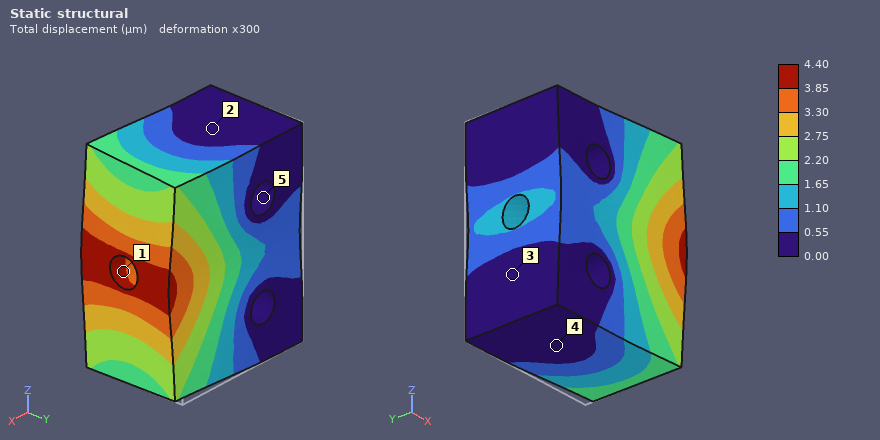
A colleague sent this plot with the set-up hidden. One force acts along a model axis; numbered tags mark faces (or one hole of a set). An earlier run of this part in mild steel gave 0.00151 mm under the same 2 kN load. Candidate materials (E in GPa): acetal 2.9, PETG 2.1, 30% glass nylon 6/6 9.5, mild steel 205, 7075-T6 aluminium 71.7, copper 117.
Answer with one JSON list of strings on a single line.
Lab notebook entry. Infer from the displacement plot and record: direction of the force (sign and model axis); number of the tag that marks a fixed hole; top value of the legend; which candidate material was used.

["-Y", "5", "4.40 µm", "7075-T6 aluminium"]
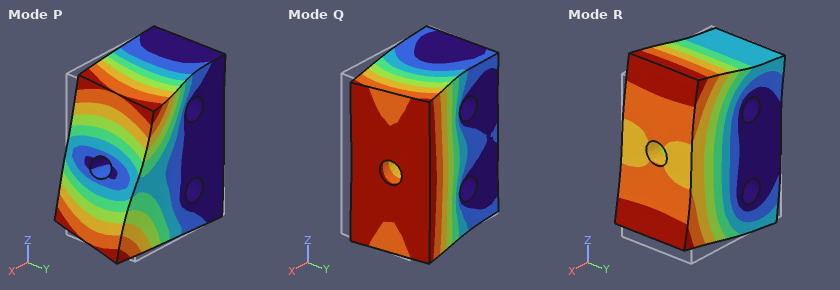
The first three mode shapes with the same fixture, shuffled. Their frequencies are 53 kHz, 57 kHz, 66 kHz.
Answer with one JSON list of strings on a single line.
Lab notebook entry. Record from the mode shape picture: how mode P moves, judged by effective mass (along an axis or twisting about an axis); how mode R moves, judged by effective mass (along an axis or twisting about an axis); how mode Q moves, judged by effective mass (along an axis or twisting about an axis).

["twisting about X", "along Z", "along Y"]
